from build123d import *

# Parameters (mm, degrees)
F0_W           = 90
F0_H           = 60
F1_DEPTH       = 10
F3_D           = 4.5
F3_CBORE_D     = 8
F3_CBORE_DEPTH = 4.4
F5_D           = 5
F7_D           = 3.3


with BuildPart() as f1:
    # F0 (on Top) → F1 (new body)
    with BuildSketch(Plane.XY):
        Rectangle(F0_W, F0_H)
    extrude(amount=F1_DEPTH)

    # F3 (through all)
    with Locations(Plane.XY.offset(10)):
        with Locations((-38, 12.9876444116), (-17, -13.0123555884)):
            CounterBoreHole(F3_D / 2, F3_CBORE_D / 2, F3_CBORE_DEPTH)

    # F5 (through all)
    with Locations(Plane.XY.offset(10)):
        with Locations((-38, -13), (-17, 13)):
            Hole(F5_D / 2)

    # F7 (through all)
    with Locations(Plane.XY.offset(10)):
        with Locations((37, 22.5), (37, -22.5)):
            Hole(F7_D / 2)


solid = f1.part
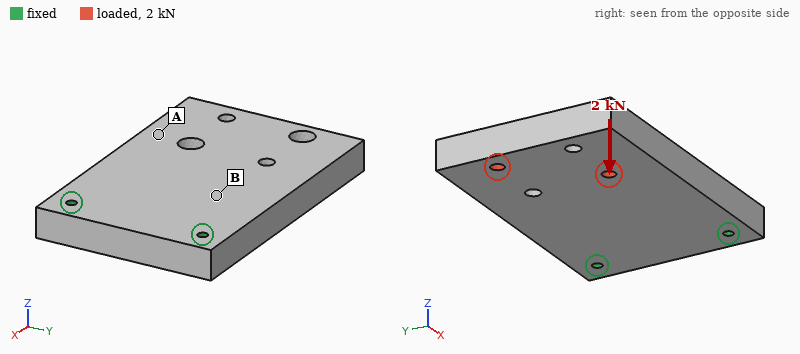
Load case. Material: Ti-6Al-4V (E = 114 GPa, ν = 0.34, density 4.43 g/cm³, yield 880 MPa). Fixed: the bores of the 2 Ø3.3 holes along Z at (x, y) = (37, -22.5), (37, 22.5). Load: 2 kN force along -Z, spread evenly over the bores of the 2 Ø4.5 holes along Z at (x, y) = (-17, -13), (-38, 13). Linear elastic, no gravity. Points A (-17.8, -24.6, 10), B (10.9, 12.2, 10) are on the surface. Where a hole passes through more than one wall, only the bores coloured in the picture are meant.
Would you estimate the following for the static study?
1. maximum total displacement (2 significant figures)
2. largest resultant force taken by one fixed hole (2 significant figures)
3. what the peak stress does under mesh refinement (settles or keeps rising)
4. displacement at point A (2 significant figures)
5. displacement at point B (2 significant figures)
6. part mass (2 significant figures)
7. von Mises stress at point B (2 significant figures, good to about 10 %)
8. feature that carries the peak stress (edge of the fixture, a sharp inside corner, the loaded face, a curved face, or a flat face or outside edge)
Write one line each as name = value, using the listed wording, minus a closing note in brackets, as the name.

maximum total displacement = 0.61 mm
largest resultant force taken by one fixed hole = 1.0 kN
what the peak stress does under mesh refinement = keeps rising
displacement at point A = 0.34 mm
displacement at point B = 0.12 mm
part mass = 230 g
von Mises stress at point B = 75 MPa
feature that carries the peak stress = edge of the fixture
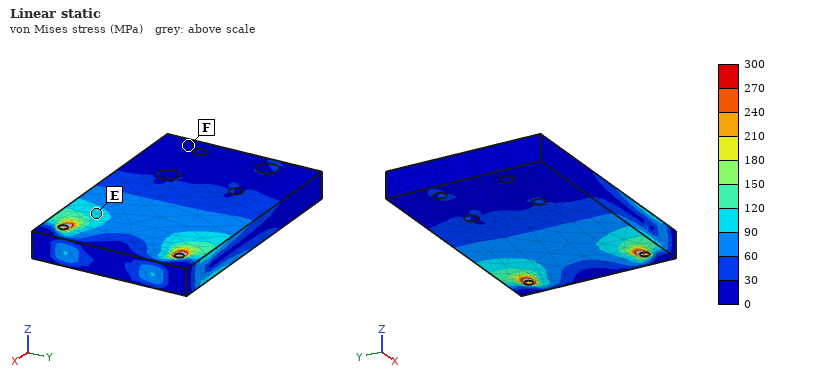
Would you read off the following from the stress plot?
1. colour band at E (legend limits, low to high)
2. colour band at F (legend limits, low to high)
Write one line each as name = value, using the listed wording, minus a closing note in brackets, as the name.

colour band at E = 90 to 120 MPa
colour band at F = 0 to 30 MPa
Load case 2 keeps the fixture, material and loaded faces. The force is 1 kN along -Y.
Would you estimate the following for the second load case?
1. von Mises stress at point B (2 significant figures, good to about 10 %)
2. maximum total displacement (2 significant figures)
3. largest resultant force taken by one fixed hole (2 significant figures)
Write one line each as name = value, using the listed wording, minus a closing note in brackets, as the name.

von Mises stress at point B = 3.4 MPa
maximum total displacement = 13 µm
largest resultant force taken by one fixed hole = 1.5 kN
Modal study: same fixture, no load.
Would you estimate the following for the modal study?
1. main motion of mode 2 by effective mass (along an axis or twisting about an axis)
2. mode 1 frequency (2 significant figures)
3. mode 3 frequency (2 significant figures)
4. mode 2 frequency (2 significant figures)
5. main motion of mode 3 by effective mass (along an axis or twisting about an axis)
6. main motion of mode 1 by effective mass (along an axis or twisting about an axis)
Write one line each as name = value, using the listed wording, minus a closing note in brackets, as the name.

main motion of mode 2 by effective mass = twisting about X
mode 1 frequency = 1100 Hz
mode 3 frequency = 5200 Hz
mode 2 frequency = 3400 Hz
main motion of mode 3 by effective mass = along Y
main motion of mode 1 by effective mass = along Z
